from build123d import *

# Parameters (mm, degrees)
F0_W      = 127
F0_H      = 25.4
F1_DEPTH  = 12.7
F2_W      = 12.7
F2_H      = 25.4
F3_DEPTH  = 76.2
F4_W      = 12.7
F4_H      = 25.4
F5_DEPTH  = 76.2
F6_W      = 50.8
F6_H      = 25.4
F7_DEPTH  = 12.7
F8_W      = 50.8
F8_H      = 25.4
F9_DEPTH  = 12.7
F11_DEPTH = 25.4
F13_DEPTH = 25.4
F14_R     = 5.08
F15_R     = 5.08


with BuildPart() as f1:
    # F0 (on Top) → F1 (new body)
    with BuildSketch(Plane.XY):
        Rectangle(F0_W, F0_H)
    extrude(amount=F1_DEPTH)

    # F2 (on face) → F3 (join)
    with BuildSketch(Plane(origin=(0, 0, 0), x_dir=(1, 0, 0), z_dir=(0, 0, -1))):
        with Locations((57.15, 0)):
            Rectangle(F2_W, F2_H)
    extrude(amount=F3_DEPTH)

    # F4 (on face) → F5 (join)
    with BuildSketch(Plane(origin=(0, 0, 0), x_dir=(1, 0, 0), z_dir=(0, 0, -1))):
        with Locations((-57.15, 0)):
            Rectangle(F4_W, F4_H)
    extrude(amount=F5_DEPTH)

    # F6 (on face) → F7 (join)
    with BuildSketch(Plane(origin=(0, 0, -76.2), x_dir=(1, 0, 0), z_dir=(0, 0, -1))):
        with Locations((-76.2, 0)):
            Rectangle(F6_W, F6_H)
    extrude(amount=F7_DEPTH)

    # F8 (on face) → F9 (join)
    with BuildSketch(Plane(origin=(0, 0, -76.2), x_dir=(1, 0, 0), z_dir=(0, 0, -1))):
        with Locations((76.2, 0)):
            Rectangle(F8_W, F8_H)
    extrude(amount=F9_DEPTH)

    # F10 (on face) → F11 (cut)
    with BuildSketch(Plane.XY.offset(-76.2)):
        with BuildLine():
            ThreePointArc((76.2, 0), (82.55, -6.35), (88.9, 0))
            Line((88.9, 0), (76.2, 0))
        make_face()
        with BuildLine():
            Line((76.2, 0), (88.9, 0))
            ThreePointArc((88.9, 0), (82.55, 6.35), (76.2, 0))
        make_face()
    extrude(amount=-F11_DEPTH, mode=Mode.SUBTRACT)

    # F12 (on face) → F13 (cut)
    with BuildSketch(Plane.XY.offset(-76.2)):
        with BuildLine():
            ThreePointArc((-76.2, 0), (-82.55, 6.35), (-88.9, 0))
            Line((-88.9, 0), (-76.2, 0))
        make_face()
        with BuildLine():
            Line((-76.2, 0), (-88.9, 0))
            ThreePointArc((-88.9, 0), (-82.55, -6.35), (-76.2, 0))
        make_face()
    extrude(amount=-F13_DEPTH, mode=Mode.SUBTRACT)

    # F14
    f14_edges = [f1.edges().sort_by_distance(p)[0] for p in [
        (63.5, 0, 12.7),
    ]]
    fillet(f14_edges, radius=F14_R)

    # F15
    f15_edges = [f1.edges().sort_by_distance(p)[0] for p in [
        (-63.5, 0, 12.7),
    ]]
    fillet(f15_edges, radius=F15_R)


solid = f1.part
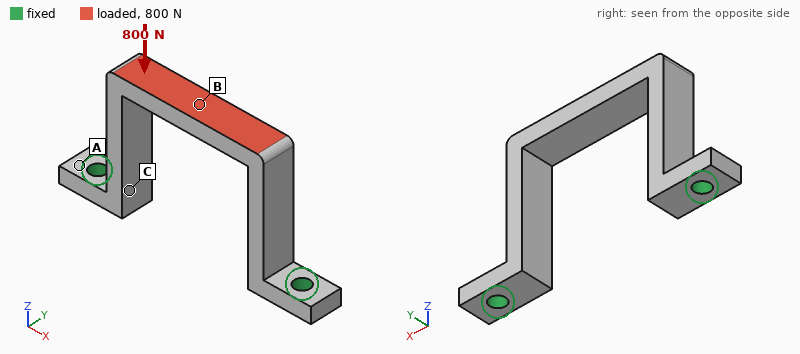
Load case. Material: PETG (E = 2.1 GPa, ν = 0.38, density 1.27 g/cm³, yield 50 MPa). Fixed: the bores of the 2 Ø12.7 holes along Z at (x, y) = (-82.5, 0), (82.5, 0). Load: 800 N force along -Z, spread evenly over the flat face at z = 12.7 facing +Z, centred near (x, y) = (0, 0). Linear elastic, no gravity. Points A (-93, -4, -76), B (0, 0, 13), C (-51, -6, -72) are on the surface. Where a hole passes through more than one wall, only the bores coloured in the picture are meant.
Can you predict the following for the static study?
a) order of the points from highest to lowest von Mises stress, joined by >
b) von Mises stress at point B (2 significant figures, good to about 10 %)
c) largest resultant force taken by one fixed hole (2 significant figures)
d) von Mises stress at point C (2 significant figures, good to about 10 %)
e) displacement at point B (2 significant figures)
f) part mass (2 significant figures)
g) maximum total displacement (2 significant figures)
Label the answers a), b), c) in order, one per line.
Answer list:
a) B > C > A
b) 7.9 MPa
c) 410 N
d) 2.4 MPa
e) 0.75 mm
f) 150 g
g) 0.78 mm
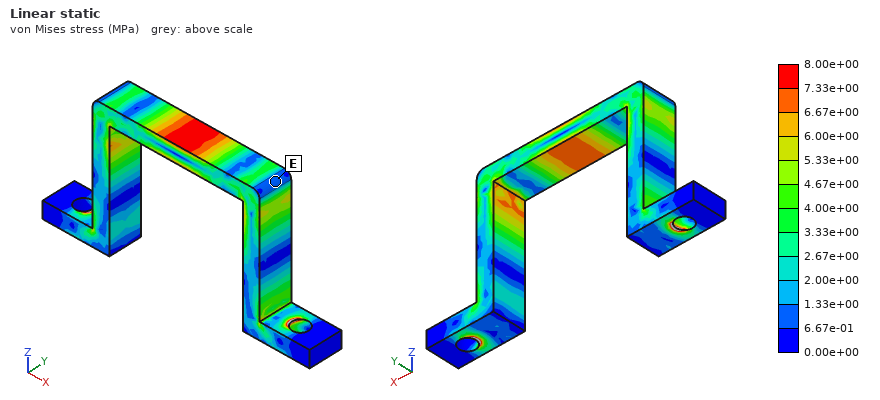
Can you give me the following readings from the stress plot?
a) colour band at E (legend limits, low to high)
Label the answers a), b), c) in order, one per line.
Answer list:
a) 6.67e-01 to 1.33e+00 MPa
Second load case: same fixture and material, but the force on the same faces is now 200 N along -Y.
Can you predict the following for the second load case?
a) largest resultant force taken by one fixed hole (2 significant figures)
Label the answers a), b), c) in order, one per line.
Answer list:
a) 100 N
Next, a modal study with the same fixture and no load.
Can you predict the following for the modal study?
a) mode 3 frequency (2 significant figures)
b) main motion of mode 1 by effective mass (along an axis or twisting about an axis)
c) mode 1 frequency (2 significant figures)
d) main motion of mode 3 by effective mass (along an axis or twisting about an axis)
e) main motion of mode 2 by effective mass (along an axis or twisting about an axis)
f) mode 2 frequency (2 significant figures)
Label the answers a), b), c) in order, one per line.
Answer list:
a) 360 Hz
b) along Y
c) 190 Hz
d) twisting about Z
e) along X
f) 240 Hz
